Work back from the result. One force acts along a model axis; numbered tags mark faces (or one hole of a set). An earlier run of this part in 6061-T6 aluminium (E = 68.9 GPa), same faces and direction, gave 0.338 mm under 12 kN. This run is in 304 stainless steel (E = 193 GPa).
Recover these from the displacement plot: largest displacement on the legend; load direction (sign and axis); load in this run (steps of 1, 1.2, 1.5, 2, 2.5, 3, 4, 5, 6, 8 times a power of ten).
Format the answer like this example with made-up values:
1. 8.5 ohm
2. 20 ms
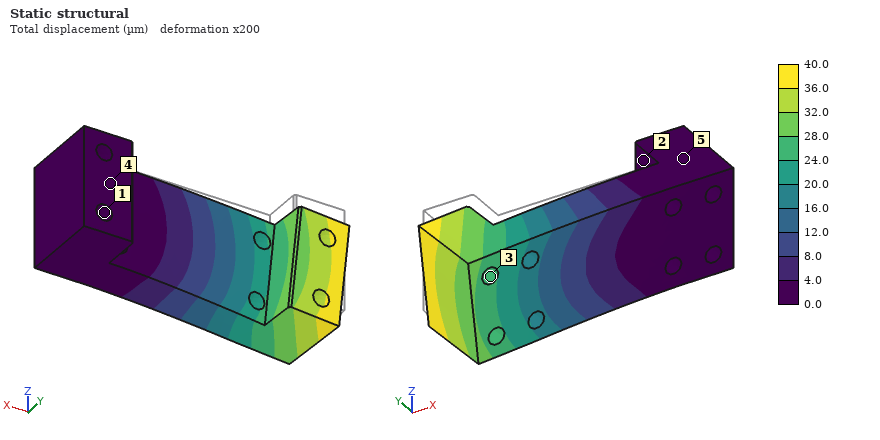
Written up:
1. 40.0 µm
2. -Z
3. 4 kN
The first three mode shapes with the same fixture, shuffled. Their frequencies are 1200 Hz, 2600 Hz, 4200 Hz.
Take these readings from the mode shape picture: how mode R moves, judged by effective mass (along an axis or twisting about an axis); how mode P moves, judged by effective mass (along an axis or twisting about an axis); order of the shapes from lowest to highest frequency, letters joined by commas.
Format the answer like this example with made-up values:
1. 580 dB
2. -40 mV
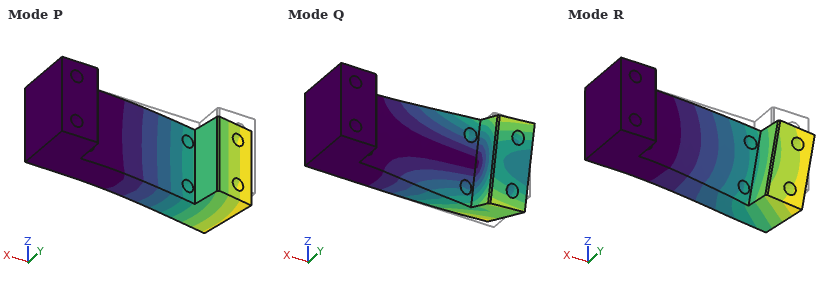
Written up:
1. along Z
2. along Y
3. P, R, Q
